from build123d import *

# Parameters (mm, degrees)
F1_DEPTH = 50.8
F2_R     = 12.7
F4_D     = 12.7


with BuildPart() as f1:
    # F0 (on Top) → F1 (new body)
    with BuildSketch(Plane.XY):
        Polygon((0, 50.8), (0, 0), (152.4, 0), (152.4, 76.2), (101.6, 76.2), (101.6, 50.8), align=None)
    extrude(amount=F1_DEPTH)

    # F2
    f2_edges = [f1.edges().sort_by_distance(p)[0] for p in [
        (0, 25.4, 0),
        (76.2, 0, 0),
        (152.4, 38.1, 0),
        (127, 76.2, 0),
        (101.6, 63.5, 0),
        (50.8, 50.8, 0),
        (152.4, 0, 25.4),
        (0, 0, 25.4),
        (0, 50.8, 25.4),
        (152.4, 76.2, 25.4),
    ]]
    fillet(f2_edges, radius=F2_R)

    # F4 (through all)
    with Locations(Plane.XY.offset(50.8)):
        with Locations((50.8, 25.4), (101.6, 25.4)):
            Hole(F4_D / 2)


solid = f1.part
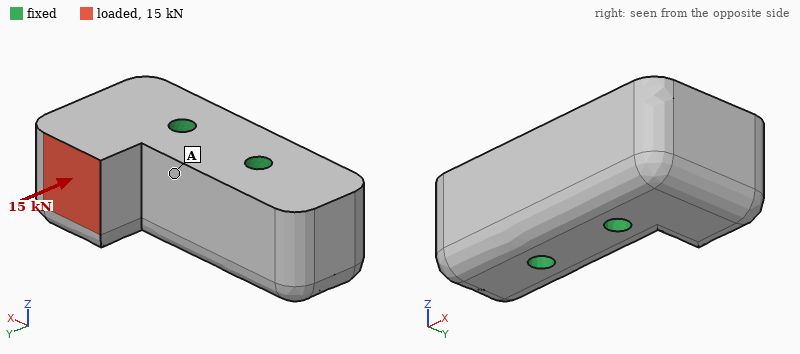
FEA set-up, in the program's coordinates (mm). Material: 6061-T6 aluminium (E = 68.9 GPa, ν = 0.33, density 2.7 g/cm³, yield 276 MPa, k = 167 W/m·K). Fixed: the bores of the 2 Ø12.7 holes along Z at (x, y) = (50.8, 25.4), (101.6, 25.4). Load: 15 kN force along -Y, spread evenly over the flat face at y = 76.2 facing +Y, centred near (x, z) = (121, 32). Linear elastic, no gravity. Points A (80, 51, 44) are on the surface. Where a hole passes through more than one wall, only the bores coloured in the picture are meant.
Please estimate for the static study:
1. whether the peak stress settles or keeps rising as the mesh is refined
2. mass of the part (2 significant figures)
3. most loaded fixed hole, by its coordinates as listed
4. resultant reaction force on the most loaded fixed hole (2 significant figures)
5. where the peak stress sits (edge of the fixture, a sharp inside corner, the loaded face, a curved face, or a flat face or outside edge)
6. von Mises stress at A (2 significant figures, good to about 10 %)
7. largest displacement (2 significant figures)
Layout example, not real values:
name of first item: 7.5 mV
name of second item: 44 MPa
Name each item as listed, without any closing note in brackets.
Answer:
whether the peak stress settles or keeps rising as the mesh is refined: keeps rising
mass of the part: 1.1 kg
most loaded fixed hole, by its coordinates as listed: (101.6, 25.4)
resultant reaction force on the most loaded fixed hole: 18 kN
where the peak stress sits: edge of the fixture
von Mises stress at A: 6.1 MPa
largest displacement: 23 µm
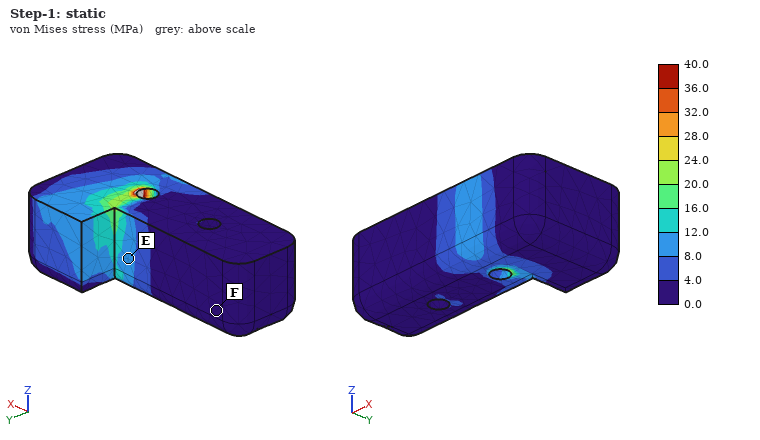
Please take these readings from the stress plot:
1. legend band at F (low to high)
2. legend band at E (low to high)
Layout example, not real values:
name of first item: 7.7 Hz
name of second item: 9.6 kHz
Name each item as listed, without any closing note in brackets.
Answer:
legend band at F: 0.0 to 4.0 MPa
legend band at E: 8.0 to 12.0 MPa
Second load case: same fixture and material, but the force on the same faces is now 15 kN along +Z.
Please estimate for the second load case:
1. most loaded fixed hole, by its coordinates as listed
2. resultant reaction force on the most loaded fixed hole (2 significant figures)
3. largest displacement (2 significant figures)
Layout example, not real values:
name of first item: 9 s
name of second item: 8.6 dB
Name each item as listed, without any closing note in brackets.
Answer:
most loaded fixed hole, by its coordinates as listed: (101.6, 25.4)
resultant reaction force on the most loaded fixed hole: 15 kN
largest displacement: 56 µm
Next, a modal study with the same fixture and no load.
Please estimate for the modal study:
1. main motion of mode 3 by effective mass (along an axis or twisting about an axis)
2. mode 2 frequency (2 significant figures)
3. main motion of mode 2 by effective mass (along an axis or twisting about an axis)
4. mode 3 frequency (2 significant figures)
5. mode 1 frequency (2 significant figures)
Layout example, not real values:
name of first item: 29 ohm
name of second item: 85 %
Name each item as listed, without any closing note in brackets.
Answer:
main motion of mode 3 by effective mass: along Y
mode 2 frequency: 7500 Hz
main motion of mode 2 by effective mass: along Z
mode 3 frequency: 8400 Hz
mode 1 frequency: 5800 Hz
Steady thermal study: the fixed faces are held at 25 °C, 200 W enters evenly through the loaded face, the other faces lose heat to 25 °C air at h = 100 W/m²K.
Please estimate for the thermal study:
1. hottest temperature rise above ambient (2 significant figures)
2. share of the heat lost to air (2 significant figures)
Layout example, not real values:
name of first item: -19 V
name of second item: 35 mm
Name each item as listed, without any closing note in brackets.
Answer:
hottest temperature rise above ambient: 31 K
share of the heat lost to air: 9.2 %
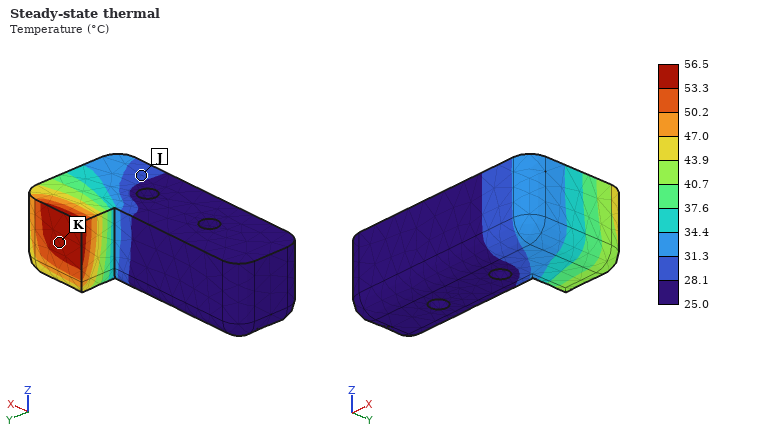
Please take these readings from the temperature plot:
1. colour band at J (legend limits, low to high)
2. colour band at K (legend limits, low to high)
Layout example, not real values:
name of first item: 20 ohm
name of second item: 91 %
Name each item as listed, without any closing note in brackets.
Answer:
colour band at J: 28.1 to 31.3 °C
colour band at K: 53.3 to 56.5 °C
